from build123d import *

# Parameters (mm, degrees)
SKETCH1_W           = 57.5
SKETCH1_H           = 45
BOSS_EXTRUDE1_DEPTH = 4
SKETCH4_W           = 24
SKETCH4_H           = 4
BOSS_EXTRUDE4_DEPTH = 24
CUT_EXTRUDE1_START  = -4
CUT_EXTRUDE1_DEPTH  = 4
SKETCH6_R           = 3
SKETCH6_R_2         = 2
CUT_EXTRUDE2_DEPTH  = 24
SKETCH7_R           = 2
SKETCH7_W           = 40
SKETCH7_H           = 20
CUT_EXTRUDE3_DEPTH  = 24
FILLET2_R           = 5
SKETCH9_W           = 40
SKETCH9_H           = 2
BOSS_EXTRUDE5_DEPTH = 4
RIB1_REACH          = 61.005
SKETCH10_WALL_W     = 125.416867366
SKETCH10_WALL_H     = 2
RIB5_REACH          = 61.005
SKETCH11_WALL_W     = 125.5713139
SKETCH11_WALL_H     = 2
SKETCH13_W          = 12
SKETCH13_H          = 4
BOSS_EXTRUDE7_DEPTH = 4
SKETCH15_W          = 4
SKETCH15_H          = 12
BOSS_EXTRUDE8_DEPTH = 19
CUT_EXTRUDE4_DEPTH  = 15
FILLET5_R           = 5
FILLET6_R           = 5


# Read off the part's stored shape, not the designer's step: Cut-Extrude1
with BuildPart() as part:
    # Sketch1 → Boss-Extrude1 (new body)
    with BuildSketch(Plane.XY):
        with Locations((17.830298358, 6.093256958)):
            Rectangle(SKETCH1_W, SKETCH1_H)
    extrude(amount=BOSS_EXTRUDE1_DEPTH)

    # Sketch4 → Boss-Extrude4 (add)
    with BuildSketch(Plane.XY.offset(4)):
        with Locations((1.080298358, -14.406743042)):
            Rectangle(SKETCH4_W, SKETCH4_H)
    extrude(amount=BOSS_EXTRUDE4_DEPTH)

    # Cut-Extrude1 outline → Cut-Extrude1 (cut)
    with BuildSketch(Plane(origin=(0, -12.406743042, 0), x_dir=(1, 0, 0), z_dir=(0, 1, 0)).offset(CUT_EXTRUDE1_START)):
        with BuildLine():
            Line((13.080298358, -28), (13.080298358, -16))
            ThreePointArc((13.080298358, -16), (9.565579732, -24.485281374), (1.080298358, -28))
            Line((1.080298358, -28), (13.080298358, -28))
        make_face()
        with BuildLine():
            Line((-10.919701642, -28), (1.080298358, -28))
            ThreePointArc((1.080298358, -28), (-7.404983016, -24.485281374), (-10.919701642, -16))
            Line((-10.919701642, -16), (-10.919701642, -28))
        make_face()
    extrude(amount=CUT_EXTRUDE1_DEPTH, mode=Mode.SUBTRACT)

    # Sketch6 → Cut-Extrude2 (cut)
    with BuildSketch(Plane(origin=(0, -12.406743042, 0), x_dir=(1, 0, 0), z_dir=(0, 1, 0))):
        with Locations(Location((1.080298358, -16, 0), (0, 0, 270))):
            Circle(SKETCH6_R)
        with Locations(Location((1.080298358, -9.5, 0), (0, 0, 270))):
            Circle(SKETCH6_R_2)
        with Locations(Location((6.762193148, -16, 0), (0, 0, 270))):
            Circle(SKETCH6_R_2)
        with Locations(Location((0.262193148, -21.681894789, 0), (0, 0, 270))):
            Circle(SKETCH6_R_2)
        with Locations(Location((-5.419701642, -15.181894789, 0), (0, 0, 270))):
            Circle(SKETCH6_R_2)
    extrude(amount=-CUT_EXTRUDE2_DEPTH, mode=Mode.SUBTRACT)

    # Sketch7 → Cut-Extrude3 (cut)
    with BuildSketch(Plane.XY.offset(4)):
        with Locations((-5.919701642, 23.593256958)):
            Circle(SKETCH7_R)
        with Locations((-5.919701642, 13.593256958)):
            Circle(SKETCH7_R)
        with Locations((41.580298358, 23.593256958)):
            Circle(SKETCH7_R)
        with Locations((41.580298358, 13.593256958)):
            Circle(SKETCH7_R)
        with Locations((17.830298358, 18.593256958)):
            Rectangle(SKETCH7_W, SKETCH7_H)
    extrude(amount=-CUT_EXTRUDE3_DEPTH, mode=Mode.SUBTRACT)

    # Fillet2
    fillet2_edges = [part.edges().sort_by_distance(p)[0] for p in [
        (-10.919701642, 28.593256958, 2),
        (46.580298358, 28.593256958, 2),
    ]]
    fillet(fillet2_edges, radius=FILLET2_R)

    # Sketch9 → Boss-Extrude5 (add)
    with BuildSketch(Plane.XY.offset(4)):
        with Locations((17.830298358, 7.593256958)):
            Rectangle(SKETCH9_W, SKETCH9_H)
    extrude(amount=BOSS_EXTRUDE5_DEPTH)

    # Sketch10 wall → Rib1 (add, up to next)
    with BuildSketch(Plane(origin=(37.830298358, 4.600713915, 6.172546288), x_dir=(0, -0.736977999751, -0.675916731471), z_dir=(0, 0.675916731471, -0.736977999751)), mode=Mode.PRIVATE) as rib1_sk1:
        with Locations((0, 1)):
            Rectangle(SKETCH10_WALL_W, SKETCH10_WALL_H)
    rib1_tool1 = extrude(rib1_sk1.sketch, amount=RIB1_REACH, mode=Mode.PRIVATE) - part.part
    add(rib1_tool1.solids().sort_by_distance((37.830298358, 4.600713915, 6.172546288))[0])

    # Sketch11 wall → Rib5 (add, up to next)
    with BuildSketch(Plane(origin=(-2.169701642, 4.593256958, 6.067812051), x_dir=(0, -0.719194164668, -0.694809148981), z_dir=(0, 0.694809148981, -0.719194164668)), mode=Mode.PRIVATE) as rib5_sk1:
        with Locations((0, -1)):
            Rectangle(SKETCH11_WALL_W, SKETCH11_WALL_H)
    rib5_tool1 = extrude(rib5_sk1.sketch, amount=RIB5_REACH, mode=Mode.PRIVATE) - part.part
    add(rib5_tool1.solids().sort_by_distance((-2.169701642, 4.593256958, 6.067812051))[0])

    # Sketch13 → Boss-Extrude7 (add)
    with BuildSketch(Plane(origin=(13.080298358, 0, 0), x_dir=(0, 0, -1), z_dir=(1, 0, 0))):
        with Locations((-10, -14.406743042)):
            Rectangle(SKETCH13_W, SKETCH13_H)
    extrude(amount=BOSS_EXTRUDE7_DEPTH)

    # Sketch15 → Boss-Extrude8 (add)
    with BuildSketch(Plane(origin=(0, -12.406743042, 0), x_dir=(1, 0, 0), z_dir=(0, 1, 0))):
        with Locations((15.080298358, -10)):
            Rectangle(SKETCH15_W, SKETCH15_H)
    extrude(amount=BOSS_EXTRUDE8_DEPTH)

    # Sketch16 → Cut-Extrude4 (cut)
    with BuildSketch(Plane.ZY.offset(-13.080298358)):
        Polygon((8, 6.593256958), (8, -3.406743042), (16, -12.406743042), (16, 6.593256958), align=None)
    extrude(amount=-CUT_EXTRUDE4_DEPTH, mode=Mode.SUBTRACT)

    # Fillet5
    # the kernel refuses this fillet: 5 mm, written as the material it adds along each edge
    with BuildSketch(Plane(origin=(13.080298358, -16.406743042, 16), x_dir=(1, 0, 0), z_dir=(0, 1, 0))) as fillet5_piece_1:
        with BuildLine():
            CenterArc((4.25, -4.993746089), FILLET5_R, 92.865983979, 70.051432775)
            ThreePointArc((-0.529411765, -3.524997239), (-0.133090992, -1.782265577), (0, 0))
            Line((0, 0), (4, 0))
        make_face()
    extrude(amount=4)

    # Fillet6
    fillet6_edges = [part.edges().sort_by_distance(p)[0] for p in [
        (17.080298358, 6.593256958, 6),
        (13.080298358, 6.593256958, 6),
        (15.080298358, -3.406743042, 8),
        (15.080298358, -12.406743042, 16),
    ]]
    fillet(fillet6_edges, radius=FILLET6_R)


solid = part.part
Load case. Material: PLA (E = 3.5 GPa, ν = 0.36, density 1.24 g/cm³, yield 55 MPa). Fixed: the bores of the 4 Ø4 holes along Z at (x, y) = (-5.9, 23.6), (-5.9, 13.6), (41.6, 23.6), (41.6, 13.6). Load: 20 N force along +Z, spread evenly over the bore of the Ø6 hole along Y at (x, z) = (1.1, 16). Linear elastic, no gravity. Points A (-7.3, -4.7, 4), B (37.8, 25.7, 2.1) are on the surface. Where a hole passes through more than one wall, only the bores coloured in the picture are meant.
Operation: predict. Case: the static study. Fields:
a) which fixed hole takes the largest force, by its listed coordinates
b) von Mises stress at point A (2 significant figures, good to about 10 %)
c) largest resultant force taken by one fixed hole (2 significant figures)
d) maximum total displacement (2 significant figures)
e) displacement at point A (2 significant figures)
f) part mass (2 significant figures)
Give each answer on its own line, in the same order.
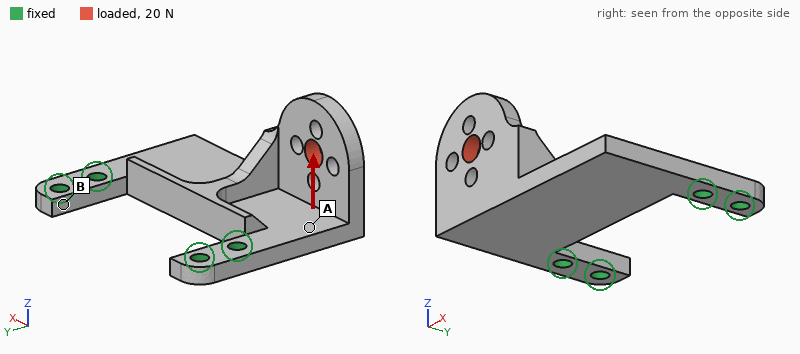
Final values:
(-5.9, 13.6)
2.3 MPa
19 N
0.57 mm
0.20 mm
12 g
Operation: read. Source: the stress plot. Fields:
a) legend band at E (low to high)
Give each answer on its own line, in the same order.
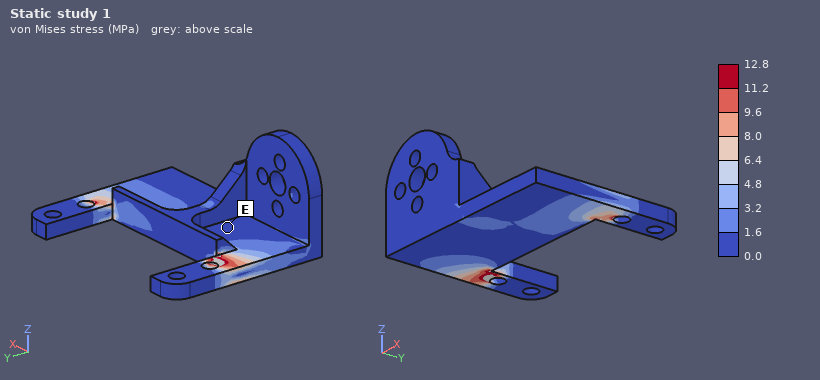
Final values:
0.0 to 1.6 MPa
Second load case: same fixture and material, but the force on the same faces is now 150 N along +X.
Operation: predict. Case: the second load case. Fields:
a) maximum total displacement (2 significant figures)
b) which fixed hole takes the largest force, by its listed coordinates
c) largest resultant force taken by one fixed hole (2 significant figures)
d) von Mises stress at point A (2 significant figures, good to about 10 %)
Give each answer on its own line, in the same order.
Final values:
0.74 mm
(41.6, 13.6)
130 N
9.8 MPa
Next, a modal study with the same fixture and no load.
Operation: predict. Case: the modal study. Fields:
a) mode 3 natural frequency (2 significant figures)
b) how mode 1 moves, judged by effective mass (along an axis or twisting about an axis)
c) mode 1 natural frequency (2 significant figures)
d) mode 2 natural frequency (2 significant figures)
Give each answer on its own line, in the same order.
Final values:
1900 Hz
along Z
490 Hz
1300 Hz
